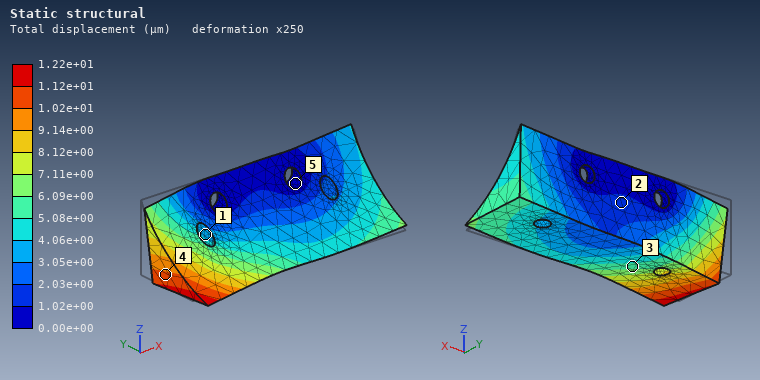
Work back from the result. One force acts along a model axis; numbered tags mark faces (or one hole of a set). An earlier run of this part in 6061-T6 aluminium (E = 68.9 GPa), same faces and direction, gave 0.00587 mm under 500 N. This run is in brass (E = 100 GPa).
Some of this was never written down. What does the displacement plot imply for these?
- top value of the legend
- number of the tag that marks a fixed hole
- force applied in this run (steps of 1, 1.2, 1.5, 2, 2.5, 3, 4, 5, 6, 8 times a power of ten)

1.22e+01 µm
5
1.5 kN
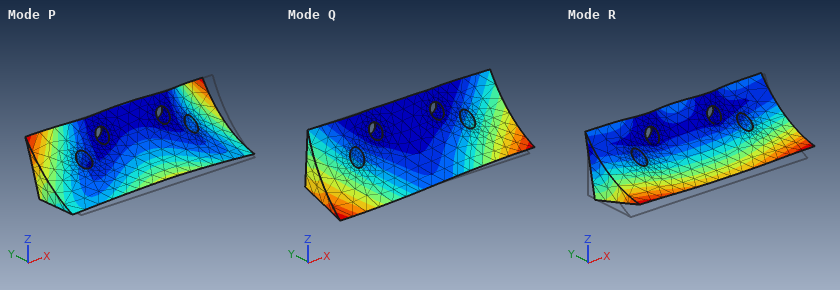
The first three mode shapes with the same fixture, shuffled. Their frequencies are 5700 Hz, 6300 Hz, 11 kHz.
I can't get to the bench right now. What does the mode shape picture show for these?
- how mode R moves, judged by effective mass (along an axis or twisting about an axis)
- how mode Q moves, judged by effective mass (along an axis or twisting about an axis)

along Y
twisting about Z
